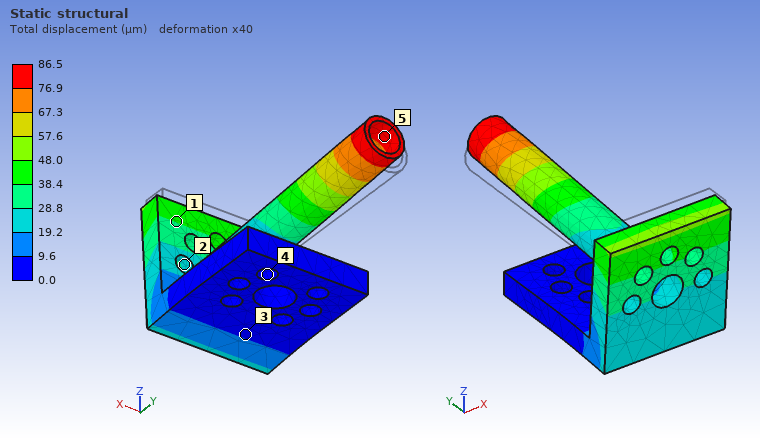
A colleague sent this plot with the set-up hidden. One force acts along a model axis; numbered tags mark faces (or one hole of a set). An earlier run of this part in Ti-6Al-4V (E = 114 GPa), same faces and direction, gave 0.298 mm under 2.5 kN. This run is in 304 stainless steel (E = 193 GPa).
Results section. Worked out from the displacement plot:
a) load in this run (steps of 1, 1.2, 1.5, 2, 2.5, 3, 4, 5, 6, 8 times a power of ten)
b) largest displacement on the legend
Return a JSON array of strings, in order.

["1.2 kN", "86.5 µm"]
